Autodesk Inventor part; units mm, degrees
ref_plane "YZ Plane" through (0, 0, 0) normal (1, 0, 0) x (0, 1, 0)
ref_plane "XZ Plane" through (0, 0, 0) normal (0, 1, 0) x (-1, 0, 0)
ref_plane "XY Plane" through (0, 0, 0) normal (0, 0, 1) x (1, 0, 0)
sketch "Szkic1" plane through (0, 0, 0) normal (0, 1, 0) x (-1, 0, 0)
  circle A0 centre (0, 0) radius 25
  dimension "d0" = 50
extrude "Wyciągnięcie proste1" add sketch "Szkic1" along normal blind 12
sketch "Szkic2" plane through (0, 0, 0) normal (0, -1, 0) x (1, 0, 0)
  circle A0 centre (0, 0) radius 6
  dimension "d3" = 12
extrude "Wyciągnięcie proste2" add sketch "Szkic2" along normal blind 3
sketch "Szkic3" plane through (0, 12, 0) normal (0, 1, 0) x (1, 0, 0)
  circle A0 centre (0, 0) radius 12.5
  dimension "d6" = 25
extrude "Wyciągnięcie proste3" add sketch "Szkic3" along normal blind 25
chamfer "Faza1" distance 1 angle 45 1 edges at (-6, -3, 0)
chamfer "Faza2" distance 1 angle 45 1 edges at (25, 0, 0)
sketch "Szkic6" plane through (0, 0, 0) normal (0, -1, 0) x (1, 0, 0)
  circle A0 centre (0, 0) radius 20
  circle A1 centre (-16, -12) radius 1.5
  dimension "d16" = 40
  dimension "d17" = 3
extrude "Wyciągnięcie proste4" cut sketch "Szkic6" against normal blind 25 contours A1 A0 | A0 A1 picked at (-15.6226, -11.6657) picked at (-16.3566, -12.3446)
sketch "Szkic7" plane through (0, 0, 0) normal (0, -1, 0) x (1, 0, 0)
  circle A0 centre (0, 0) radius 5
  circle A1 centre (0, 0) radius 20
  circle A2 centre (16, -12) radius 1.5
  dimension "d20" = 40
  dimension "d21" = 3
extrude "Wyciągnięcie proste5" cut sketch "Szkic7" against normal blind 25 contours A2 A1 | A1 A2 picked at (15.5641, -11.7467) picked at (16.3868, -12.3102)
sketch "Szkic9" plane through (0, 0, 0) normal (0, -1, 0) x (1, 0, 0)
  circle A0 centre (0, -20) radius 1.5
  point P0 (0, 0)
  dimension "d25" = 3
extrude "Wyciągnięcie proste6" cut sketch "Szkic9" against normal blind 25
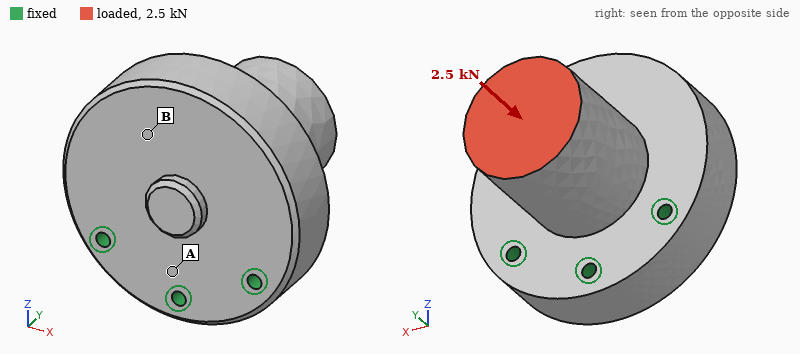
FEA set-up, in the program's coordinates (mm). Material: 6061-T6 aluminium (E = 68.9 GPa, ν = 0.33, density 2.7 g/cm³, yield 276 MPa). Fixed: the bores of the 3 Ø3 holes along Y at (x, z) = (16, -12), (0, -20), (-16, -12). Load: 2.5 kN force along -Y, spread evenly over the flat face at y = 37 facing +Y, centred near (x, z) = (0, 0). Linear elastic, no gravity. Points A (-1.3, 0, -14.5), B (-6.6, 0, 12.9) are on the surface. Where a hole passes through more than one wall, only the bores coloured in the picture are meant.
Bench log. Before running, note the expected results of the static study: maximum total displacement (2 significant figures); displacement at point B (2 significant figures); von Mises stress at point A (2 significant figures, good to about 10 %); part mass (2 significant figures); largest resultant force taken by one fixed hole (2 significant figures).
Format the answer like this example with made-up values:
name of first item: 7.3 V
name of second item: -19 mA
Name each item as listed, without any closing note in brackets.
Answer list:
maximum total displacement: 30 µm
displacement at point B: 20 µm
von Mises stress at point A: 20 MPa
part mass: 97 g
largest resultant force taken by one fixed hole: 1.2 kN
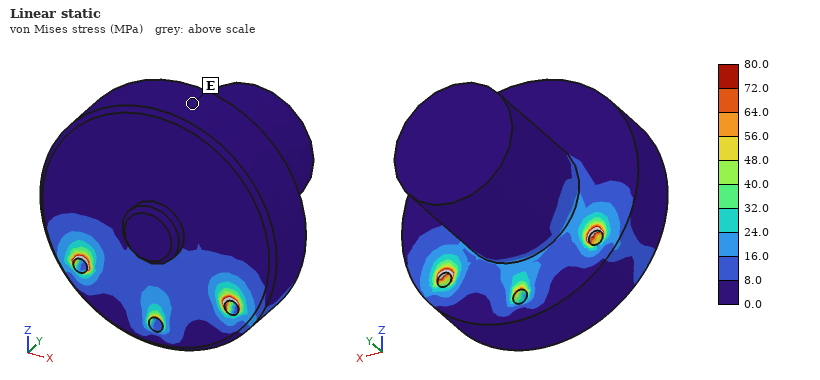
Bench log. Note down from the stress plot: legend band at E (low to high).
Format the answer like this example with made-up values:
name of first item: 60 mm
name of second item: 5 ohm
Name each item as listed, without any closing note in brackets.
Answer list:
legend band at E: 0.0 to 8.0 MPa
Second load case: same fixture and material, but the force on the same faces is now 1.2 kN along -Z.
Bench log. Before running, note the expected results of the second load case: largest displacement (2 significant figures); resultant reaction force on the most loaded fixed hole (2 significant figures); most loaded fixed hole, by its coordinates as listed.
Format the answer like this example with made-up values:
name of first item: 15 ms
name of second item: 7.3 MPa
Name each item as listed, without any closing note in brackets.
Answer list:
largest displacement: 46 µm
resultant reaction force on the most loaded fixed hole: 1.1 kN
most loaded fixed hole, by its coordinates as listed: (0, -20)
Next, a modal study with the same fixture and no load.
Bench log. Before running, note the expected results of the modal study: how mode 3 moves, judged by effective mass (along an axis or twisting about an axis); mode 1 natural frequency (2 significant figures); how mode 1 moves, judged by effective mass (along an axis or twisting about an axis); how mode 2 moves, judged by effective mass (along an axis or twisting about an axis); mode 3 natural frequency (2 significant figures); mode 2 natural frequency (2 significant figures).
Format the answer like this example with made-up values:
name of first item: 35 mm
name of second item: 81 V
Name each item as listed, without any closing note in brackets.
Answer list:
how mode 3 moves, judged by effective mass: along X
mode 1 natural frequency: 5100 Hz
how mode 1 moves, judged by effective mass: along Y
how mode 2 moves, judged by effective mass: along X
mode 3 natural frequency: 15 kHz
mode 2 natural frequency: 10 kHz
